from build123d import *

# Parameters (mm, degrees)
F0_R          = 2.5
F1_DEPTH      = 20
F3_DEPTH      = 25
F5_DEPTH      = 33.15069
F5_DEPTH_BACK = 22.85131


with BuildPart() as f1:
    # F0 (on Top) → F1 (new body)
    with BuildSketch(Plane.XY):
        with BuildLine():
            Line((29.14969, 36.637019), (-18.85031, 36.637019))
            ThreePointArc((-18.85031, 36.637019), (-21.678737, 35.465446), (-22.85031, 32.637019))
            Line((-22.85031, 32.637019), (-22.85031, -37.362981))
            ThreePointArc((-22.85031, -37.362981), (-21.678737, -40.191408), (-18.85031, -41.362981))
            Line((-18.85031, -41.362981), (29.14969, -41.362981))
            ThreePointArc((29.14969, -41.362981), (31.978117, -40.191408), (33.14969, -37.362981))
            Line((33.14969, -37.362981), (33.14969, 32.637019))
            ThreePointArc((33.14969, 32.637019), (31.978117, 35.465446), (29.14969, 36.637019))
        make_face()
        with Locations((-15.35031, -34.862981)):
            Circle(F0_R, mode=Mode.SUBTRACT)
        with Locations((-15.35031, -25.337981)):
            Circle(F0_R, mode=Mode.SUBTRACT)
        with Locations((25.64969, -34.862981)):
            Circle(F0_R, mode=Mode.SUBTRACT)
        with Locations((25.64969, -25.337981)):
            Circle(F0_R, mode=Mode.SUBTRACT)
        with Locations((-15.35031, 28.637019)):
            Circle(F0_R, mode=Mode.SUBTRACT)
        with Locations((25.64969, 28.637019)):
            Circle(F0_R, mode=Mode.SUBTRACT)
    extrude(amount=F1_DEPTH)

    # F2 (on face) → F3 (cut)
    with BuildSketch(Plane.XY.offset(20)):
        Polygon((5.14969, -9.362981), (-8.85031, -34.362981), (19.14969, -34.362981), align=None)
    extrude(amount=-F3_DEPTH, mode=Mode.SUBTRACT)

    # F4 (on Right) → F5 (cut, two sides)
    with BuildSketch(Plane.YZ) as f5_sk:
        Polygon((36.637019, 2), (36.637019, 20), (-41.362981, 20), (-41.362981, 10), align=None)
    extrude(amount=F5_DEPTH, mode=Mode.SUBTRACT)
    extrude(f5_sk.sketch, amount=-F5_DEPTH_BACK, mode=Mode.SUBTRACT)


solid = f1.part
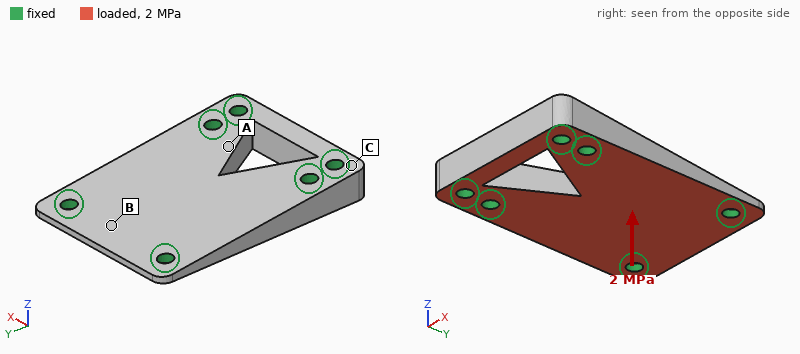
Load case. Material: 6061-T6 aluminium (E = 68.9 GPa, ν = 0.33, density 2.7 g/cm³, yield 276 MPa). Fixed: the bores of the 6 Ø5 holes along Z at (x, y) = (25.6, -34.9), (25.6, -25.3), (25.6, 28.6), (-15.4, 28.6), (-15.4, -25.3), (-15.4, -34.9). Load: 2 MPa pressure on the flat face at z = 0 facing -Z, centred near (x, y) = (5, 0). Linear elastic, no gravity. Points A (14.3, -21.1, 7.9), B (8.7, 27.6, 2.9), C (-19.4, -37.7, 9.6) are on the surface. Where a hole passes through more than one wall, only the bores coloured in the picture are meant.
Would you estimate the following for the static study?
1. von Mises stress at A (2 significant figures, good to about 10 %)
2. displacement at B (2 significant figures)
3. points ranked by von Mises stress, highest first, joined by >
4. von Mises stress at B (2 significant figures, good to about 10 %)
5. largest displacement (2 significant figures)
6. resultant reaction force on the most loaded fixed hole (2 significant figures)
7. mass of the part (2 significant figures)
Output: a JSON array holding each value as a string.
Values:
["41 MPa", "0.092 mm", "B > A > C", "81 MPa", "0.11 mm", "2.1 kN", "60 g"]
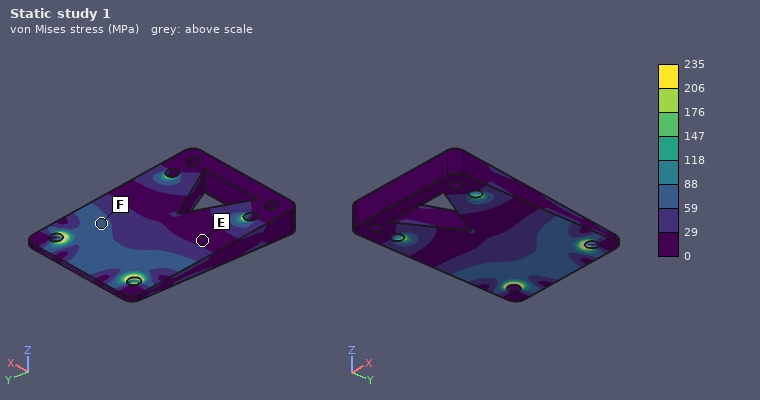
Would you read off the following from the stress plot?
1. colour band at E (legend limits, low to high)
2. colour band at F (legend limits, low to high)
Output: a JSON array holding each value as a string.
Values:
["0 to 29 MPa", "59 to 88 MPa"]
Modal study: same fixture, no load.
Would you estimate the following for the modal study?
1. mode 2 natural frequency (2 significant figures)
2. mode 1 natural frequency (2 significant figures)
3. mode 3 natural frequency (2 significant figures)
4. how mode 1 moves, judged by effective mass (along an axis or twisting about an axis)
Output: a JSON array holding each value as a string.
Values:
["11 kHz", "7600 Hz", "11 kHz", "along Z"]
